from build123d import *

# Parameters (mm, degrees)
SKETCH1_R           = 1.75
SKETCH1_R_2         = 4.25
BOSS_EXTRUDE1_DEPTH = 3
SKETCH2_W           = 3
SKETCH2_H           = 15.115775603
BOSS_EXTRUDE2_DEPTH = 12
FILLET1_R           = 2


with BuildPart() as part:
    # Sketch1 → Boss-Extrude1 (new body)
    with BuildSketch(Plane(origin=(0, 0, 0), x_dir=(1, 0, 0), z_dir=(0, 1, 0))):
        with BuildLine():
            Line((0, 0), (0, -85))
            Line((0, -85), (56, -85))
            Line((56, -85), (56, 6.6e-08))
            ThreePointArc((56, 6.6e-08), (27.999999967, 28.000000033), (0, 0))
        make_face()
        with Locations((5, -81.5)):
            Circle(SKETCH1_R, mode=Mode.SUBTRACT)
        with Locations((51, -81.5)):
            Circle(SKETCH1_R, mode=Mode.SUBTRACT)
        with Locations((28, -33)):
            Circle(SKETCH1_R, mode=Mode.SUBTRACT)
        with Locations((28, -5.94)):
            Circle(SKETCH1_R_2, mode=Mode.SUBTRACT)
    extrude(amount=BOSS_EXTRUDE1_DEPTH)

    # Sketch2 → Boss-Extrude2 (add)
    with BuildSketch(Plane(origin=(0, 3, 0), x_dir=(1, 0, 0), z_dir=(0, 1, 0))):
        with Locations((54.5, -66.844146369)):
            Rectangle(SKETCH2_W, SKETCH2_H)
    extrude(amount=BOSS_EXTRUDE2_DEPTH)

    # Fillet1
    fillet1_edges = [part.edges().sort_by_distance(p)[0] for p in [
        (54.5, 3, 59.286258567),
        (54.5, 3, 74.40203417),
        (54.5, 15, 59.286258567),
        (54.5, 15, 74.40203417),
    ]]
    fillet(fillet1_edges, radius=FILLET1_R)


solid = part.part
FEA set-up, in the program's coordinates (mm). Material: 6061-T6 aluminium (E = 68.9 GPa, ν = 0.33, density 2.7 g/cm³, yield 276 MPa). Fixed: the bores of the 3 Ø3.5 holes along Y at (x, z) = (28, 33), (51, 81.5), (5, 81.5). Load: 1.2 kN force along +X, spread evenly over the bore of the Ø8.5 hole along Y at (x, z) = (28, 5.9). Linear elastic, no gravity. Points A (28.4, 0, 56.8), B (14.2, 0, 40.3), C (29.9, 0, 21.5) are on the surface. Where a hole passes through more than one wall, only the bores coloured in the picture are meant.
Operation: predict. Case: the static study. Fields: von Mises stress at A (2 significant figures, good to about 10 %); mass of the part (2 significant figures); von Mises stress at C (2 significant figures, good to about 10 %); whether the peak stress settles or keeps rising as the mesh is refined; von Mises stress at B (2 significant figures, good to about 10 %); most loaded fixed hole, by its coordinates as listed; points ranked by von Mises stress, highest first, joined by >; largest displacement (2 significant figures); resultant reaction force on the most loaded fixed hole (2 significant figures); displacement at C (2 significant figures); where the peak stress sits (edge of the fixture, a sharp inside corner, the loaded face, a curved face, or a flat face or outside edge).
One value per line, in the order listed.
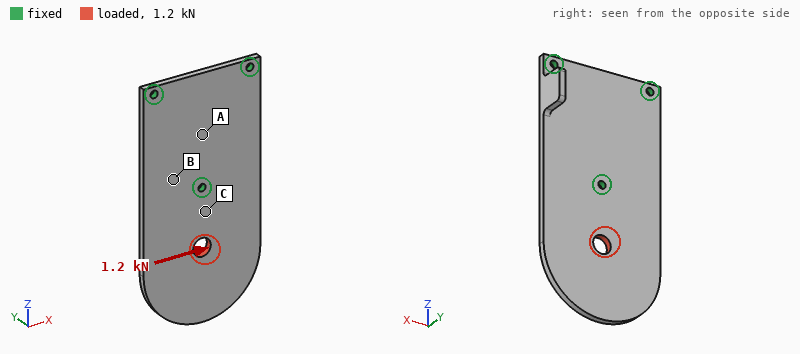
5.4 MPa
49 g
17 MPa
keeps rising
10 MPa
(28, 33)
C > B > A
43 µm
1.6 kN
11 µm
edge of the fixture
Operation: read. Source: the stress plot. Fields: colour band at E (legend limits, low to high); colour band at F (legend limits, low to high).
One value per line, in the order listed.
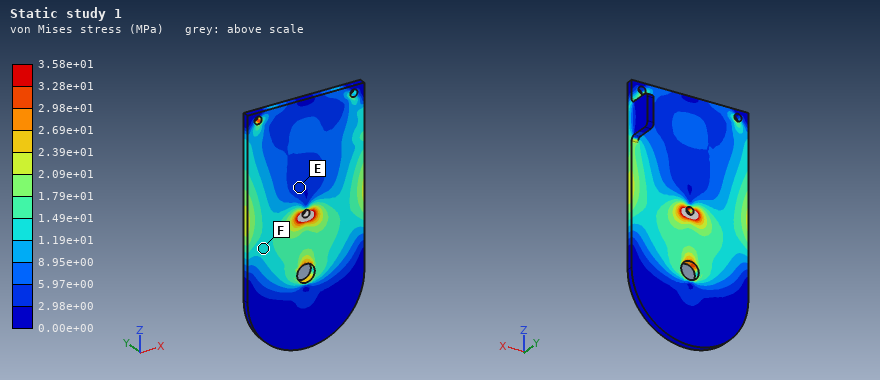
2.98e+00 to 5.97e+00 MPa
1.19e+01 to 1.49e+01 MPa
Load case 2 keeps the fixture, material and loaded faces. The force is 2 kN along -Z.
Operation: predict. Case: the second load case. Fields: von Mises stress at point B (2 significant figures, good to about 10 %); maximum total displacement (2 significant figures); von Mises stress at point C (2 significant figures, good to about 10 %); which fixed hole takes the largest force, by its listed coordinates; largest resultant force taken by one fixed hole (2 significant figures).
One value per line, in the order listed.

6.9 MPa
13 µm
26 MPa
(28, 33)
1.4 kN
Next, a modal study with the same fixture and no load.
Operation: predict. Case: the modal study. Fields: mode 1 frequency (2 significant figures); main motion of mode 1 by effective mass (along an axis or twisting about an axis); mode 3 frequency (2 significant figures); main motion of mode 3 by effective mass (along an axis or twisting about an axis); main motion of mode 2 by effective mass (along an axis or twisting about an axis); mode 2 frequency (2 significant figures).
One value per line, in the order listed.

710 Hz
along Y
3200 Hz
along Y
twisting about Z
1500 Hz
